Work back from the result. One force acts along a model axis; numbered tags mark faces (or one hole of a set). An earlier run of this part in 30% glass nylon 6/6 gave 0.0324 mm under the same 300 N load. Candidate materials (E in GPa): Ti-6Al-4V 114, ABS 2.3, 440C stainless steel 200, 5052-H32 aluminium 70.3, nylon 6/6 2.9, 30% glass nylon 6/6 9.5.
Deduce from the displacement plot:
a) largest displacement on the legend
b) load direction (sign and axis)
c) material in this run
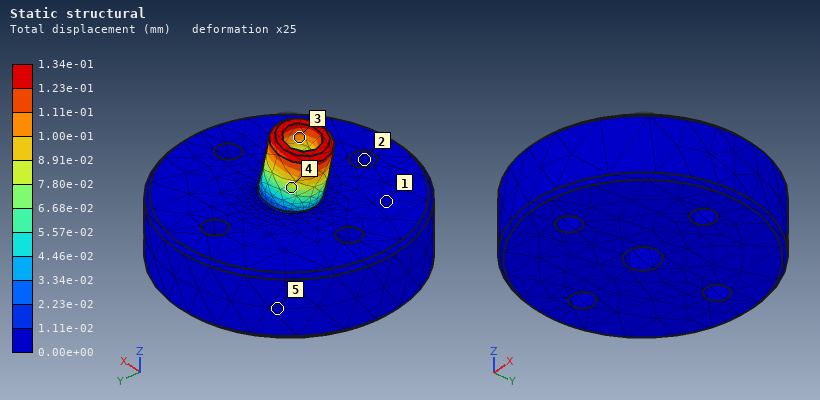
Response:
1.34e-01 mm
-X
ABS
